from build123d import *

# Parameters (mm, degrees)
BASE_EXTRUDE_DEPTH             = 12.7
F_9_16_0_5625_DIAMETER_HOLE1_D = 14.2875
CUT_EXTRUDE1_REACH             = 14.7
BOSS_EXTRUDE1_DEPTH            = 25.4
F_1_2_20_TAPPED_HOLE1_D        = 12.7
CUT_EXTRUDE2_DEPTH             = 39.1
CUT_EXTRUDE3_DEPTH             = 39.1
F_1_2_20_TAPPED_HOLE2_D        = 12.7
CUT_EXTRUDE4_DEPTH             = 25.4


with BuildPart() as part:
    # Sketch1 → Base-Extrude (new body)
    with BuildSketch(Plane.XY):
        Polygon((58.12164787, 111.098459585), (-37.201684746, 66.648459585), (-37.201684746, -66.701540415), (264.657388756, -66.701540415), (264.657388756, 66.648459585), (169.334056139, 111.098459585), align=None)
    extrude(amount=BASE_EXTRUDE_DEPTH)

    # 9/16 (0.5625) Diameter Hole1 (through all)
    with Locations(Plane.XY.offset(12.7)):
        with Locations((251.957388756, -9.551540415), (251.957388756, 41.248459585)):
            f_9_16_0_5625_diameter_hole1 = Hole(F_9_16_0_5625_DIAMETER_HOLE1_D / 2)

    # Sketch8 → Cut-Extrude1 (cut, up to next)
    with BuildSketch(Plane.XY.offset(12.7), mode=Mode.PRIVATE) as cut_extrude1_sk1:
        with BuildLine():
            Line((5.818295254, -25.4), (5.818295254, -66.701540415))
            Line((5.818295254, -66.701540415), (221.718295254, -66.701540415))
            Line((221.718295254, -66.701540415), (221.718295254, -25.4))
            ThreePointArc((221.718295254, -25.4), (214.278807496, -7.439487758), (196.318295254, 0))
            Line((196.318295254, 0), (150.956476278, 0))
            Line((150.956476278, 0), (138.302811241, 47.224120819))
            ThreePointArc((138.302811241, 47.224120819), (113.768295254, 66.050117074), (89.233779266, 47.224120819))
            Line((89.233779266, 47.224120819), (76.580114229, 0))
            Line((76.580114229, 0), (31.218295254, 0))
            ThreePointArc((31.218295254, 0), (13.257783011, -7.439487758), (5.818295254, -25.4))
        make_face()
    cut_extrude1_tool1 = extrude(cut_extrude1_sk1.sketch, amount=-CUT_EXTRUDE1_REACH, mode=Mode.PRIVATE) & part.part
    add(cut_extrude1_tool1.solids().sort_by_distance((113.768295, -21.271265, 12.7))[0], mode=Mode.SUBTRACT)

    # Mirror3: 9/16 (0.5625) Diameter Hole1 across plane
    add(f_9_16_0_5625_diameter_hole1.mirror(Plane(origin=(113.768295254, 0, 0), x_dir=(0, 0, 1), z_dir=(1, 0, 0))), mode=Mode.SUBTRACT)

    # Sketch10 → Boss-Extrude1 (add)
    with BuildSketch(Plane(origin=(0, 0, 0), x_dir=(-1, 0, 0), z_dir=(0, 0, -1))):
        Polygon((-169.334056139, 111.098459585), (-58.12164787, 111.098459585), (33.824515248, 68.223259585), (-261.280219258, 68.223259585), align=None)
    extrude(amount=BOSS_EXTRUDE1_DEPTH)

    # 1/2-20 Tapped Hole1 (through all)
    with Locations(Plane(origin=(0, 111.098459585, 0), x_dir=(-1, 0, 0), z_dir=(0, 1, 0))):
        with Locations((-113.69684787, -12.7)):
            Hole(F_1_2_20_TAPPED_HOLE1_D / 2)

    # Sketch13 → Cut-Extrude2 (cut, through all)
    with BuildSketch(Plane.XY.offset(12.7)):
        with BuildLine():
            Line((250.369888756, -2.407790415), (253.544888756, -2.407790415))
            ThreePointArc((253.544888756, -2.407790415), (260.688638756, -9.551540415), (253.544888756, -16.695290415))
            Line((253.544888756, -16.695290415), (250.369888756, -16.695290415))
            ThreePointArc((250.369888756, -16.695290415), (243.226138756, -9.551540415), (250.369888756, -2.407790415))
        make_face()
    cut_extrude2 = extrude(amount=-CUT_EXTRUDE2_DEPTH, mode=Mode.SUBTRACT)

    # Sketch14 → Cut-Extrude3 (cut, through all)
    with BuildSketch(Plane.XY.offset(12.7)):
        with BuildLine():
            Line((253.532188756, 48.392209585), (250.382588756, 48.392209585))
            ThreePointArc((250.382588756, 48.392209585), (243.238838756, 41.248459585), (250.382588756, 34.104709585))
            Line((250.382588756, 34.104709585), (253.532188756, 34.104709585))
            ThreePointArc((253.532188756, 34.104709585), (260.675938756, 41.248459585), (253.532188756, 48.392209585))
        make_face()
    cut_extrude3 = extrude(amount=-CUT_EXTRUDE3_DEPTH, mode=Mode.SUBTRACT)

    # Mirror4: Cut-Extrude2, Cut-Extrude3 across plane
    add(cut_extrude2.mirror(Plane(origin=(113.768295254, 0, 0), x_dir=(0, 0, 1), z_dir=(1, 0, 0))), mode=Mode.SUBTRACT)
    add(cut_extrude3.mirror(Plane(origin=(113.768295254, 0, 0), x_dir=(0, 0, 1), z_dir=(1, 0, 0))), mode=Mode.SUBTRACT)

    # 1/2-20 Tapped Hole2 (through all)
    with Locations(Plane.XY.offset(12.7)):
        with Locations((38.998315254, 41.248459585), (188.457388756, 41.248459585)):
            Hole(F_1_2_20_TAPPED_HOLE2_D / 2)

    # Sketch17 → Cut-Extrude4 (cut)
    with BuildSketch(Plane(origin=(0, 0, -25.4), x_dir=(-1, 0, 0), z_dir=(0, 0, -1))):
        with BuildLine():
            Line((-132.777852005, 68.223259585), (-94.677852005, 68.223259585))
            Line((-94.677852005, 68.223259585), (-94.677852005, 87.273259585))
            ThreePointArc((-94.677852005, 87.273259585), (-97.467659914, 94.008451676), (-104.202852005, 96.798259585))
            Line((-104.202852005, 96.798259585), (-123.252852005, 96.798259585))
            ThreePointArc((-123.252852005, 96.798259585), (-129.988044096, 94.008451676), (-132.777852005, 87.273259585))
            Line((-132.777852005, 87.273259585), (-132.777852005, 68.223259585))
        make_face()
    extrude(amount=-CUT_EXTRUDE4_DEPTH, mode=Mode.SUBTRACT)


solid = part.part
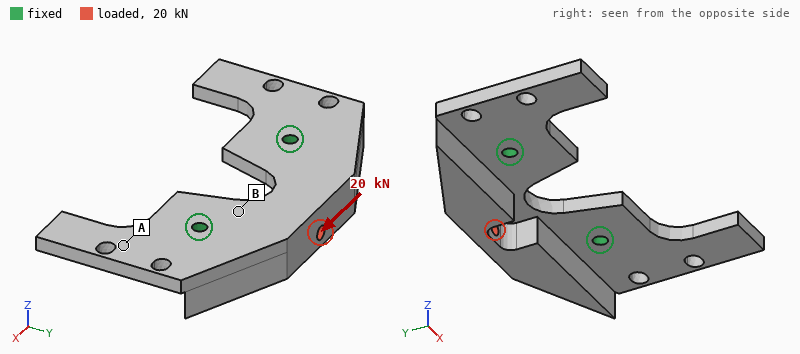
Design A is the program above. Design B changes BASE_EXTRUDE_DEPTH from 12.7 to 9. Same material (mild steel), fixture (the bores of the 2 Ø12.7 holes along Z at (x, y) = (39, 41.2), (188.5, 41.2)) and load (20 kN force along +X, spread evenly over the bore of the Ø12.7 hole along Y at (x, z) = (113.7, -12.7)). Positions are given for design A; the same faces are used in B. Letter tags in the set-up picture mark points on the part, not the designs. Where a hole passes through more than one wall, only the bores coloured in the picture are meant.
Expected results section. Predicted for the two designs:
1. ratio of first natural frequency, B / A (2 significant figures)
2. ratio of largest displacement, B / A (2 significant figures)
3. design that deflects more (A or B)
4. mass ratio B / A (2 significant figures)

0.73
1.6
B
0.81
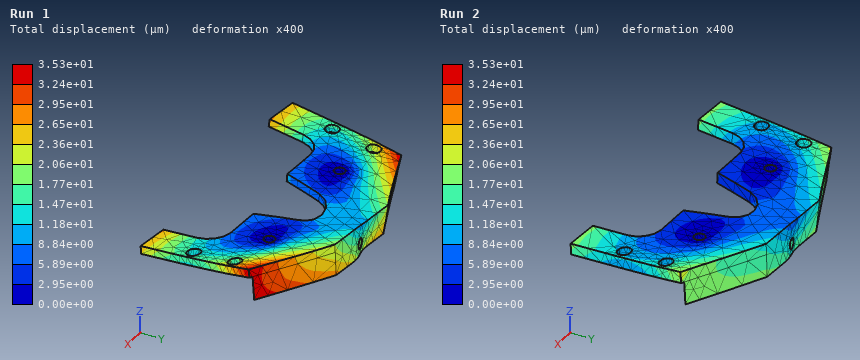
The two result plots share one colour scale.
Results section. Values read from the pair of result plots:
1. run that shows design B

Run 1
